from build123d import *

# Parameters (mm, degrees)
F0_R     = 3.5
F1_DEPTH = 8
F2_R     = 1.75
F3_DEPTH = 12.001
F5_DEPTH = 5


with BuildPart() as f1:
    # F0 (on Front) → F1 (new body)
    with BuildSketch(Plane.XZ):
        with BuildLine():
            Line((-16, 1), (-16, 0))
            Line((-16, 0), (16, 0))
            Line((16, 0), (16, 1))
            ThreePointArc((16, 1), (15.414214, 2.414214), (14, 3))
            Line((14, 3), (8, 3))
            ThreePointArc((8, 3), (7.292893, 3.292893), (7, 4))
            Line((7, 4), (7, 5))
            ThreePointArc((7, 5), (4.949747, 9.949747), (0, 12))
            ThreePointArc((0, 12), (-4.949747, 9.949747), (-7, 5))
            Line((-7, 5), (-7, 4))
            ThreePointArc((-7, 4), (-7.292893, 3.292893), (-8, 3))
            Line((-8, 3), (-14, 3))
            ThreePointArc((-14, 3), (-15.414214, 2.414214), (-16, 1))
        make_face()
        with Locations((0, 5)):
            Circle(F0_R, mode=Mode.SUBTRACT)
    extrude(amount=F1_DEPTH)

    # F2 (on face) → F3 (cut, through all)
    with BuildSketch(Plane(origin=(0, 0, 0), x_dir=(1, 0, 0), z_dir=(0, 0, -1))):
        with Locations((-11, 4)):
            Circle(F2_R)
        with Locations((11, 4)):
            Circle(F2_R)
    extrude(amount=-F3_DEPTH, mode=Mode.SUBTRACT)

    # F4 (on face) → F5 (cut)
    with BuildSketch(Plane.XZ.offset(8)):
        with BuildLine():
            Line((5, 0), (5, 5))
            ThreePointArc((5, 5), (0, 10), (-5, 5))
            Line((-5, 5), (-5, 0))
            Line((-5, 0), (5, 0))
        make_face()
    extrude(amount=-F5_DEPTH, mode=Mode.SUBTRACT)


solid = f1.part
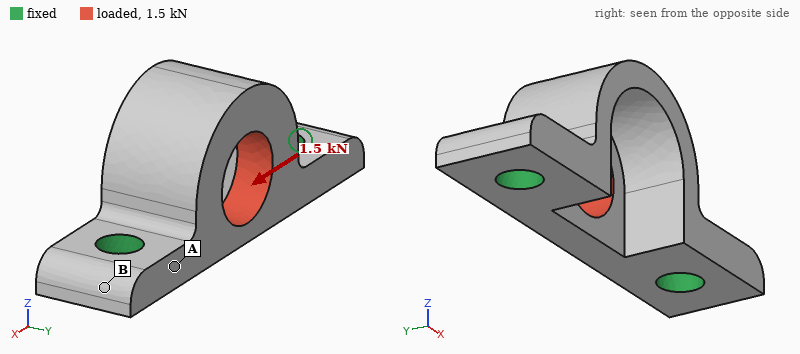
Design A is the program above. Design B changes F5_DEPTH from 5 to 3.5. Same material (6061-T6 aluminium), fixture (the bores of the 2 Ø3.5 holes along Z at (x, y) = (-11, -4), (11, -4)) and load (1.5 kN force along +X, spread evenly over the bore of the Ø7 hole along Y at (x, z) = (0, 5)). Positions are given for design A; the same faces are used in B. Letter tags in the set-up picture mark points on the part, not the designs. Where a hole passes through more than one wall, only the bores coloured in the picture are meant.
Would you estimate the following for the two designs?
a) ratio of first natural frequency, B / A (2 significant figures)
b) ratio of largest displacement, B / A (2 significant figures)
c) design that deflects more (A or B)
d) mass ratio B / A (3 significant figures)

0.98
0.76
A
1.08
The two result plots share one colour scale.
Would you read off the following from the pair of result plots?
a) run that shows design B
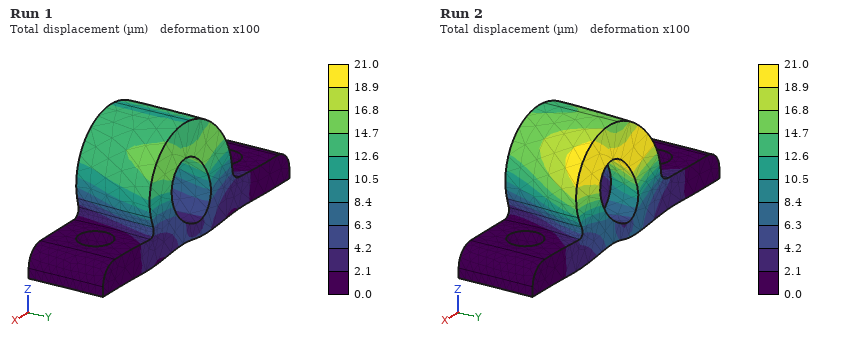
Run 1
